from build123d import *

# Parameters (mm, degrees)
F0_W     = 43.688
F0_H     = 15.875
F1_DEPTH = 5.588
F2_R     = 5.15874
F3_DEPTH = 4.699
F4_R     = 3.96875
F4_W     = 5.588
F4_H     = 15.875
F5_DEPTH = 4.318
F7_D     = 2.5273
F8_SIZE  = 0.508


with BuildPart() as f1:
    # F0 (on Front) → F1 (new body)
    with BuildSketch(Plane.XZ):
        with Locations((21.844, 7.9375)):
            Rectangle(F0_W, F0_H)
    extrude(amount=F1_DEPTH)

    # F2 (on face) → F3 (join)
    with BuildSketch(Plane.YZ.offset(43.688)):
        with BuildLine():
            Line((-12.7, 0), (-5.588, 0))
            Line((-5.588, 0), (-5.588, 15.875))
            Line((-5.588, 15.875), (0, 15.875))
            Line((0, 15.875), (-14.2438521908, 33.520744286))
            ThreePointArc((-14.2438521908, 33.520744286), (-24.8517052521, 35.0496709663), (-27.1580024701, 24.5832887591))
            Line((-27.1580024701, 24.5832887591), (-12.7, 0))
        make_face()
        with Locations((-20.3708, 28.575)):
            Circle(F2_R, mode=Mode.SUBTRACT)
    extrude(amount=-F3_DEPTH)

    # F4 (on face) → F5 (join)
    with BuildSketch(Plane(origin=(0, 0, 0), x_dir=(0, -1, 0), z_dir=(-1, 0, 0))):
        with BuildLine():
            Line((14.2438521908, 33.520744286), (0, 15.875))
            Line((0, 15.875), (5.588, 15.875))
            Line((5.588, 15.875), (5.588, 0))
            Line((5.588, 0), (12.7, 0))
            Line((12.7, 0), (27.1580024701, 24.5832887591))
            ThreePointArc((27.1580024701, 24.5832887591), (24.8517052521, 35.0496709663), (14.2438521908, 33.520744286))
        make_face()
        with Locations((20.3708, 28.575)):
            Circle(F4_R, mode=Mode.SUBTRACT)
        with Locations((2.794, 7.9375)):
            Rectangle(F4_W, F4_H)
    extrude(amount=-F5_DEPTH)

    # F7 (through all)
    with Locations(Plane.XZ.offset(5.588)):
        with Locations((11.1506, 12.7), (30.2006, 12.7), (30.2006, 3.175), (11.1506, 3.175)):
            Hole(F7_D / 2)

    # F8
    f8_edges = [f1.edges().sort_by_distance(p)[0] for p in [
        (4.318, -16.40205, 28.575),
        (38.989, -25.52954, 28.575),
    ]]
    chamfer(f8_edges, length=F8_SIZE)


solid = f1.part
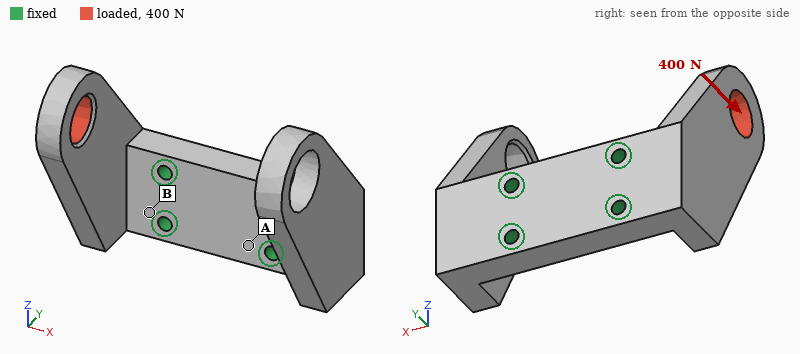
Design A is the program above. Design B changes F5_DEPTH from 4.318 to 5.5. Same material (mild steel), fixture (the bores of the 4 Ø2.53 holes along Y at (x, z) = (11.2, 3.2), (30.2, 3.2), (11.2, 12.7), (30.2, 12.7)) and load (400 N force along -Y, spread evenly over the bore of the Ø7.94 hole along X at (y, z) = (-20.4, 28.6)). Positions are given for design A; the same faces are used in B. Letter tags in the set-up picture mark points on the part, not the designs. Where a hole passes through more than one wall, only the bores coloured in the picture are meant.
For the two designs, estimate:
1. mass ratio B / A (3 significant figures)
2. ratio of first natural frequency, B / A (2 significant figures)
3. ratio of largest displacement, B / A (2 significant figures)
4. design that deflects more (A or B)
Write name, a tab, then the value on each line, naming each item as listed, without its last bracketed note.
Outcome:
mass ratio B / A	1.07
ratio of first natural frequency, B / A	1.1
ratio of largest displacement, B / A	0.79
design that deflects more	A
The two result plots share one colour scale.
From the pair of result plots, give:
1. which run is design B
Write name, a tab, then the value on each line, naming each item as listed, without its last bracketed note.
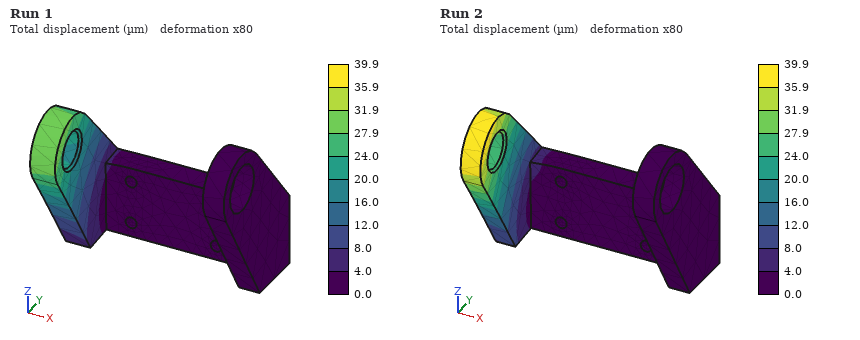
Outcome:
which run is design B	Run 1
